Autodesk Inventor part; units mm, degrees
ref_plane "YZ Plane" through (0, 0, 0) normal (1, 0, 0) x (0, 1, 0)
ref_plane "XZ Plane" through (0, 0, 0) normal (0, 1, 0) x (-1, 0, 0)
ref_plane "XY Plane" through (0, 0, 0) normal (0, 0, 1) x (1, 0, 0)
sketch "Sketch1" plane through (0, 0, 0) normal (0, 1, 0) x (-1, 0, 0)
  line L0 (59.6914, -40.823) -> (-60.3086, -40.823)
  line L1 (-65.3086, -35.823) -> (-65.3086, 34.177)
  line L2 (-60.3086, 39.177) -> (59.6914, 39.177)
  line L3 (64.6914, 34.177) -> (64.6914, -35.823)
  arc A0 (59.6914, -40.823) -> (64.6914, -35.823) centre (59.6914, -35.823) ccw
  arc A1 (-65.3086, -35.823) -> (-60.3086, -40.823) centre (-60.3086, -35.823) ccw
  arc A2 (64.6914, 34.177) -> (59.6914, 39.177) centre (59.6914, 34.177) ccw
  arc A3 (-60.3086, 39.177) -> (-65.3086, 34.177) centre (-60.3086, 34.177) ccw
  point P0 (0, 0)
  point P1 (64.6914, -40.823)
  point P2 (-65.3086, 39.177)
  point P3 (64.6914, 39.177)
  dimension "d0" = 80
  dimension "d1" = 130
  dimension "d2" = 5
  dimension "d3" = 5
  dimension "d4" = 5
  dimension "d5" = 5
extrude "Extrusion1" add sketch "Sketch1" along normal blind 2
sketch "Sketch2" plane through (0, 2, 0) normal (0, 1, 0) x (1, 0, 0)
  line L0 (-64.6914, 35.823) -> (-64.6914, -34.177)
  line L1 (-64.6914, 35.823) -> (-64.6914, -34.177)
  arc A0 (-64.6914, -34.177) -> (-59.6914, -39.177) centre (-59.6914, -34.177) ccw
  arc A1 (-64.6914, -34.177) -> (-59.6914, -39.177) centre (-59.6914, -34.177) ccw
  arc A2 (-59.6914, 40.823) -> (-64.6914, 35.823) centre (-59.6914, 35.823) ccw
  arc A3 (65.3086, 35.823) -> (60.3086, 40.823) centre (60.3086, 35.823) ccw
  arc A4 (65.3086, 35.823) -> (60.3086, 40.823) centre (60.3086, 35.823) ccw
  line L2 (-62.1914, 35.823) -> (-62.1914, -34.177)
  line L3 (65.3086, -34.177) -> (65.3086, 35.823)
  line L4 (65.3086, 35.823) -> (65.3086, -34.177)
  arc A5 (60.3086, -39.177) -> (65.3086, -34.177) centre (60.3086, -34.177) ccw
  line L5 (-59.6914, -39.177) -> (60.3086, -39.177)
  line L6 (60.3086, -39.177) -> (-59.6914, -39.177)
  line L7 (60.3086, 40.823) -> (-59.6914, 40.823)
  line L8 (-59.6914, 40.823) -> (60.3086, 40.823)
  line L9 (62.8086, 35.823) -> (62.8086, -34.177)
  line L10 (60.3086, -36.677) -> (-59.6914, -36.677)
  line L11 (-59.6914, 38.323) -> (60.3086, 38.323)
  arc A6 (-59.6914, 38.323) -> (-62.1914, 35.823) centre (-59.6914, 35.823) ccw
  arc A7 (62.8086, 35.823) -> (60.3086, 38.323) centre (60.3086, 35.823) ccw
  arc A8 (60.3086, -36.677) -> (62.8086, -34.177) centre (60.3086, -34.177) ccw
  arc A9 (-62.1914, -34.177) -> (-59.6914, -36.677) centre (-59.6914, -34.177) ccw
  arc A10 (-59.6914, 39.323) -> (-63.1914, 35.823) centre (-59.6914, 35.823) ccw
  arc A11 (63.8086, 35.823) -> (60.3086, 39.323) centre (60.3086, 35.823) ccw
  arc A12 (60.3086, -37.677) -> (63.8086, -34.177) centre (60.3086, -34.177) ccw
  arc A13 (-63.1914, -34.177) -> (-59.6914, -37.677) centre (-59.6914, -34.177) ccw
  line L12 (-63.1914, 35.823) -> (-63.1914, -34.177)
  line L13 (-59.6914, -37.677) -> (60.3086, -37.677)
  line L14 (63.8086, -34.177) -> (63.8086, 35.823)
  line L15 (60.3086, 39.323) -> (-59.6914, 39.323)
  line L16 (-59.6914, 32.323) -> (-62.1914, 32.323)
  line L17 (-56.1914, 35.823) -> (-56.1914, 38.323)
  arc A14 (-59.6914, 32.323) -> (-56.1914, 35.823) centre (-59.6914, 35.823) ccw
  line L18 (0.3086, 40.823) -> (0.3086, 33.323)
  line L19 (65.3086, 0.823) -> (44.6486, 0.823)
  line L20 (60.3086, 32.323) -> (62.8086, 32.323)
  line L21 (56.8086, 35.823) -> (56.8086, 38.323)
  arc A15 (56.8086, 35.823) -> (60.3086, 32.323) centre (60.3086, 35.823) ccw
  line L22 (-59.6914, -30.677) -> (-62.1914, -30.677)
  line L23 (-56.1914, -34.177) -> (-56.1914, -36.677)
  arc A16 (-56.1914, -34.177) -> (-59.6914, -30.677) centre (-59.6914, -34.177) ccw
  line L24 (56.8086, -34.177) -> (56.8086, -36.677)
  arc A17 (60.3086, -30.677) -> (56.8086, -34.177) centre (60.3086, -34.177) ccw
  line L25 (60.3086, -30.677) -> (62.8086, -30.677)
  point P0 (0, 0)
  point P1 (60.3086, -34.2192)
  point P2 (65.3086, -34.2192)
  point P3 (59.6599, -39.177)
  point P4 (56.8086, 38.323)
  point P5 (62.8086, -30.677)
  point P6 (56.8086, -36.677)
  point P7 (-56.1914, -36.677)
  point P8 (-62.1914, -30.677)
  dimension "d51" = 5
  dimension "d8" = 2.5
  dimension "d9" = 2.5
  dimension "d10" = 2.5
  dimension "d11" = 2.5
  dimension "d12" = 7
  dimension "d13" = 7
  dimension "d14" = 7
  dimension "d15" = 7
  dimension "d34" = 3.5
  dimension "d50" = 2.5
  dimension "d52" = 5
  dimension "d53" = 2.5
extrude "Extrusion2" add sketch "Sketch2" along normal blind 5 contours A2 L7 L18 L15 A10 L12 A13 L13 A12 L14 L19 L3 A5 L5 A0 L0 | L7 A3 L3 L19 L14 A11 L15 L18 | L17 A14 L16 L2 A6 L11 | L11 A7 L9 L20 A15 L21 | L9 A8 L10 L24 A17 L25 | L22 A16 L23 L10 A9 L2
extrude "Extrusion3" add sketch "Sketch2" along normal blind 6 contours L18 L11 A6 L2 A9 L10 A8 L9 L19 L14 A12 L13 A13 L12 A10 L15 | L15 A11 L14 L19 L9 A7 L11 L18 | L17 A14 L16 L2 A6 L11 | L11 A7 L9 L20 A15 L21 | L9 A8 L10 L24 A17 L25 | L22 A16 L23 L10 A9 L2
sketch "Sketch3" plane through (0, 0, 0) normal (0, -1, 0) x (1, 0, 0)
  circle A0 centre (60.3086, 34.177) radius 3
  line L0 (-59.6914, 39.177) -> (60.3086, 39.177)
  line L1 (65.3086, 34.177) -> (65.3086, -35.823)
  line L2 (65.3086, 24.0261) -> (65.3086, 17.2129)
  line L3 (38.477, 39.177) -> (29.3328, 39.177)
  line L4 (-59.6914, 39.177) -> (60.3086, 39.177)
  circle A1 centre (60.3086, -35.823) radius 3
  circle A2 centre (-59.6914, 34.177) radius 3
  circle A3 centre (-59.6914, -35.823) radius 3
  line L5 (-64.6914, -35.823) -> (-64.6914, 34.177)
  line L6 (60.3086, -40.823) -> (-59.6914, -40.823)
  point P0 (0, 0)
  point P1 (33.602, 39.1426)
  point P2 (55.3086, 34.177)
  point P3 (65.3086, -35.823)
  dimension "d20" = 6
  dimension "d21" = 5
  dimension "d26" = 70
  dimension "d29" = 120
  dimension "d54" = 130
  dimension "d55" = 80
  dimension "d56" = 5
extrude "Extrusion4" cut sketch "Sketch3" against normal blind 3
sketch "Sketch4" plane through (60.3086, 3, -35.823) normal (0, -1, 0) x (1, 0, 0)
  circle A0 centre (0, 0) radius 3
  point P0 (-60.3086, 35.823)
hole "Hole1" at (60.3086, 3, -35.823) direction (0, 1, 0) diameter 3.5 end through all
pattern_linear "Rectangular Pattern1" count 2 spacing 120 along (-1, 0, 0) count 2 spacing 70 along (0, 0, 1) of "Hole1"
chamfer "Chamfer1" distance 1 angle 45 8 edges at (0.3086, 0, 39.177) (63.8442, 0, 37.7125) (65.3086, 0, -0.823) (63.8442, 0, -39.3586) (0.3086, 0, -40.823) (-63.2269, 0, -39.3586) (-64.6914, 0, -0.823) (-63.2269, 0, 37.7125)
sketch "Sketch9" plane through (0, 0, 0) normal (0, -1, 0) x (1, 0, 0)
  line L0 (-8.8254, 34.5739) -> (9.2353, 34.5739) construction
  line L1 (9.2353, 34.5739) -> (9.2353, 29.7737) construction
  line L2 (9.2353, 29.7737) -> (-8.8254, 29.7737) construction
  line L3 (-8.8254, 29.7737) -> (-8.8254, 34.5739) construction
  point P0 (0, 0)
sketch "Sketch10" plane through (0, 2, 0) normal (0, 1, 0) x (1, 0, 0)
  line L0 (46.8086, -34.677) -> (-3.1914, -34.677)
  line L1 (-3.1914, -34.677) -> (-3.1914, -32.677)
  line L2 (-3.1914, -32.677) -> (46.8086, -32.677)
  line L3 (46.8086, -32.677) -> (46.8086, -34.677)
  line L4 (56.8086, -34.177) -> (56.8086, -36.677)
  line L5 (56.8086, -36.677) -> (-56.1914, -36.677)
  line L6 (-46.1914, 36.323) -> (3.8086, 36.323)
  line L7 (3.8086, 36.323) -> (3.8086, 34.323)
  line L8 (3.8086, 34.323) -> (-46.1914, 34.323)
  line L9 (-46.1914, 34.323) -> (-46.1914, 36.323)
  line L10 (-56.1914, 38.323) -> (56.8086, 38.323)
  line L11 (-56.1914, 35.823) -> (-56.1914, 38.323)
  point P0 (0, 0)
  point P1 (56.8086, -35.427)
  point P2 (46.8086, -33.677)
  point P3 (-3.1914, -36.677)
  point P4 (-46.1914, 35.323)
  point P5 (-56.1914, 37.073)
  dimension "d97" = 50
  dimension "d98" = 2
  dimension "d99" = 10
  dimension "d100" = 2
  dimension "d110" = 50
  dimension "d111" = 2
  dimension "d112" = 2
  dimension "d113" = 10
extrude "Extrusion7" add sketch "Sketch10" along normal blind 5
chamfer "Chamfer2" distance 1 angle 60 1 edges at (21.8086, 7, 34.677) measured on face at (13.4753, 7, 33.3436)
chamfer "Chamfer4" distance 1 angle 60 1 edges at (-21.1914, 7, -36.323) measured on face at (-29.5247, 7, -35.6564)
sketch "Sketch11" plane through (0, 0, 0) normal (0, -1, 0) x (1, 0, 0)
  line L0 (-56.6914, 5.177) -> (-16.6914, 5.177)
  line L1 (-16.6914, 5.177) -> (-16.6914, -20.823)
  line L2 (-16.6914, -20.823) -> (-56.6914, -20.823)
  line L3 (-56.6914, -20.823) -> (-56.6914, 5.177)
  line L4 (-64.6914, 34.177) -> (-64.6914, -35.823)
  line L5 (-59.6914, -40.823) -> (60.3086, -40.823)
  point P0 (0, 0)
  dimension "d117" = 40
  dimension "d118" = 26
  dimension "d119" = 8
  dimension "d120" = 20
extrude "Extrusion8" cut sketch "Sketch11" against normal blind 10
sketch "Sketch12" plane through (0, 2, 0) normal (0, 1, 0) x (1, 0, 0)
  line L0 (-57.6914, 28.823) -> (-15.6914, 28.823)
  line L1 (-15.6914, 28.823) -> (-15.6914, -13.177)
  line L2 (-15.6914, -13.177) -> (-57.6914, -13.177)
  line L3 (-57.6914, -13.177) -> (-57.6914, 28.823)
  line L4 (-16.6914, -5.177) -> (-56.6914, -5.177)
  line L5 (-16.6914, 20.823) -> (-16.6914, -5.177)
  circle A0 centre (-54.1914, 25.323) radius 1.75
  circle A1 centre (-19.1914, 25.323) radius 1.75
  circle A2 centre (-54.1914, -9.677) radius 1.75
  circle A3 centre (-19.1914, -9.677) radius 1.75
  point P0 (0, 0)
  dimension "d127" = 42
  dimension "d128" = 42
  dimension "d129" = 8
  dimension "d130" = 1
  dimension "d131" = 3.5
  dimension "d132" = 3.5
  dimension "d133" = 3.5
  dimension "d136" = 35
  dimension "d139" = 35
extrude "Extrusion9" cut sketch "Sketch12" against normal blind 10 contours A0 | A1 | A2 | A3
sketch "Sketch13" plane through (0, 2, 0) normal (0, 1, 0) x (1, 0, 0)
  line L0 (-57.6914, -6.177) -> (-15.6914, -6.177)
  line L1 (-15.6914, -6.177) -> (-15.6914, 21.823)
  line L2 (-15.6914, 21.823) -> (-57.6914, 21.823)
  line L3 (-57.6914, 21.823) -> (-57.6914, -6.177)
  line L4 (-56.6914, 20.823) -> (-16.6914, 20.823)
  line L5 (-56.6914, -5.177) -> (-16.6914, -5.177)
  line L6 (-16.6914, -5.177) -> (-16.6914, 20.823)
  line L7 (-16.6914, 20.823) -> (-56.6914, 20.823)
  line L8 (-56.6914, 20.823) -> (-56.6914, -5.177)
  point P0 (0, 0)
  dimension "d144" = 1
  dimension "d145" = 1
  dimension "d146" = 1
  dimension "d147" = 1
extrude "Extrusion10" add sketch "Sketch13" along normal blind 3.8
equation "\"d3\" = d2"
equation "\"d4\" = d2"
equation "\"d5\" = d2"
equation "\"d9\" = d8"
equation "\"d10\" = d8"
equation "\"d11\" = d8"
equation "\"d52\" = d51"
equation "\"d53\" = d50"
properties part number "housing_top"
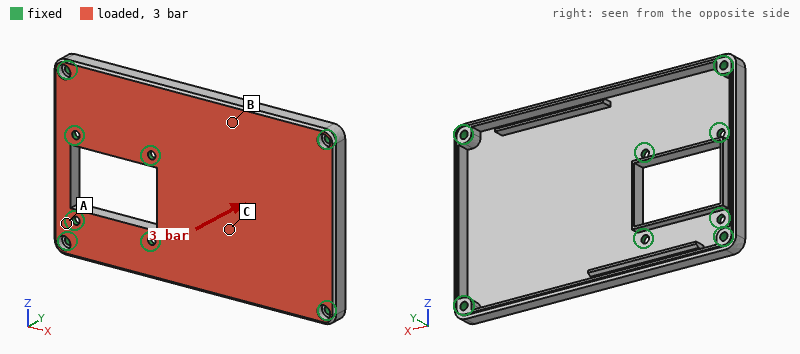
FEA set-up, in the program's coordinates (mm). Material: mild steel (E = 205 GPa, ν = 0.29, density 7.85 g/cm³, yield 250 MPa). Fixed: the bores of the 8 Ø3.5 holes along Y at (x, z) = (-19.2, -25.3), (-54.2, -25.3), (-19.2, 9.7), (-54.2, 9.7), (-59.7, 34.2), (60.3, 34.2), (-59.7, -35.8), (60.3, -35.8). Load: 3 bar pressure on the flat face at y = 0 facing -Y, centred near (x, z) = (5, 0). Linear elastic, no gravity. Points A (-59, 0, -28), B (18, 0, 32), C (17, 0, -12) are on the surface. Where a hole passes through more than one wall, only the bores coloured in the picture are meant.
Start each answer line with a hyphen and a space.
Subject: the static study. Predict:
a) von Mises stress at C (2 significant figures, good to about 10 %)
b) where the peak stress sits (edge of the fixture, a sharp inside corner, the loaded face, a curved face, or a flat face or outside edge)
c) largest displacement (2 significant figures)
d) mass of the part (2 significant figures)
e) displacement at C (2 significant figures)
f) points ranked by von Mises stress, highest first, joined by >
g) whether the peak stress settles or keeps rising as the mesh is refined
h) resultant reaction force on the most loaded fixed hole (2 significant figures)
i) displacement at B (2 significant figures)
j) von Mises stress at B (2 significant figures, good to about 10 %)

- 86 MPa
- edge of the fixture
- 0.21 mm
- 200 g
- 0.18 mm
- C > B > A
- keeps rising
- 860 N
- 0.095 mm
- 60 MPa
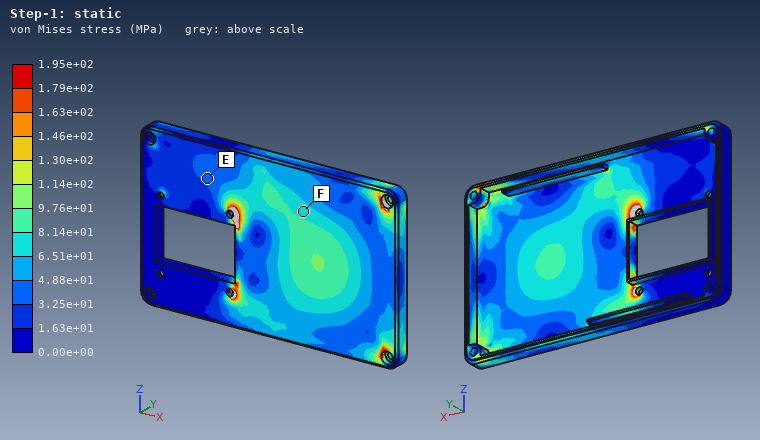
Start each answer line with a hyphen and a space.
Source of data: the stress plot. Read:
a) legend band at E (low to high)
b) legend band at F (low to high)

- 3.25e+01 to 4.88e+01 MPa
- 6.51e+01 to 8.14e+01 MPa
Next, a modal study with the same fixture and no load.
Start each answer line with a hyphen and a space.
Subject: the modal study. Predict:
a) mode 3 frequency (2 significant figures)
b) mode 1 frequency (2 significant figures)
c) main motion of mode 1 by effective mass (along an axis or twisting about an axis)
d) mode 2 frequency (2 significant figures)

- 3500 Hz
- 1900 Hz
- along Y
- 2700 Hz
